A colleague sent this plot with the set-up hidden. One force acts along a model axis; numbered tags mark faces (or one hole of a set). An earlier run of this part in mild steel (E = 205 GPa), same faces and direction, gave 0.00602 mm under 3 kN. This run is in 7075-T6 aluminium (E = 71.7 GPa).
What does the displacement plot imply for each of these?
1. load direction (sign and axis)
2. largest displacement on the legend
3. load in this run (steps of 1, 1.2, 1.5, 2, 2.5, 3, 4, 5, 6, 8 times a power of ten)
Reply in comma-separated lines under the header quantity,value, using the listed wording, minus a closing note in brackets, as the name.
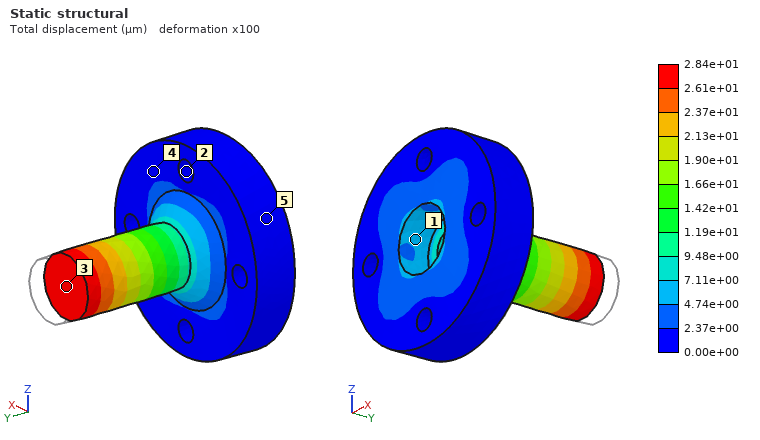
quantity,value
load direction,-Y
largest displacement on the legend,2.84e+01 µm
load in this run,5 kN
